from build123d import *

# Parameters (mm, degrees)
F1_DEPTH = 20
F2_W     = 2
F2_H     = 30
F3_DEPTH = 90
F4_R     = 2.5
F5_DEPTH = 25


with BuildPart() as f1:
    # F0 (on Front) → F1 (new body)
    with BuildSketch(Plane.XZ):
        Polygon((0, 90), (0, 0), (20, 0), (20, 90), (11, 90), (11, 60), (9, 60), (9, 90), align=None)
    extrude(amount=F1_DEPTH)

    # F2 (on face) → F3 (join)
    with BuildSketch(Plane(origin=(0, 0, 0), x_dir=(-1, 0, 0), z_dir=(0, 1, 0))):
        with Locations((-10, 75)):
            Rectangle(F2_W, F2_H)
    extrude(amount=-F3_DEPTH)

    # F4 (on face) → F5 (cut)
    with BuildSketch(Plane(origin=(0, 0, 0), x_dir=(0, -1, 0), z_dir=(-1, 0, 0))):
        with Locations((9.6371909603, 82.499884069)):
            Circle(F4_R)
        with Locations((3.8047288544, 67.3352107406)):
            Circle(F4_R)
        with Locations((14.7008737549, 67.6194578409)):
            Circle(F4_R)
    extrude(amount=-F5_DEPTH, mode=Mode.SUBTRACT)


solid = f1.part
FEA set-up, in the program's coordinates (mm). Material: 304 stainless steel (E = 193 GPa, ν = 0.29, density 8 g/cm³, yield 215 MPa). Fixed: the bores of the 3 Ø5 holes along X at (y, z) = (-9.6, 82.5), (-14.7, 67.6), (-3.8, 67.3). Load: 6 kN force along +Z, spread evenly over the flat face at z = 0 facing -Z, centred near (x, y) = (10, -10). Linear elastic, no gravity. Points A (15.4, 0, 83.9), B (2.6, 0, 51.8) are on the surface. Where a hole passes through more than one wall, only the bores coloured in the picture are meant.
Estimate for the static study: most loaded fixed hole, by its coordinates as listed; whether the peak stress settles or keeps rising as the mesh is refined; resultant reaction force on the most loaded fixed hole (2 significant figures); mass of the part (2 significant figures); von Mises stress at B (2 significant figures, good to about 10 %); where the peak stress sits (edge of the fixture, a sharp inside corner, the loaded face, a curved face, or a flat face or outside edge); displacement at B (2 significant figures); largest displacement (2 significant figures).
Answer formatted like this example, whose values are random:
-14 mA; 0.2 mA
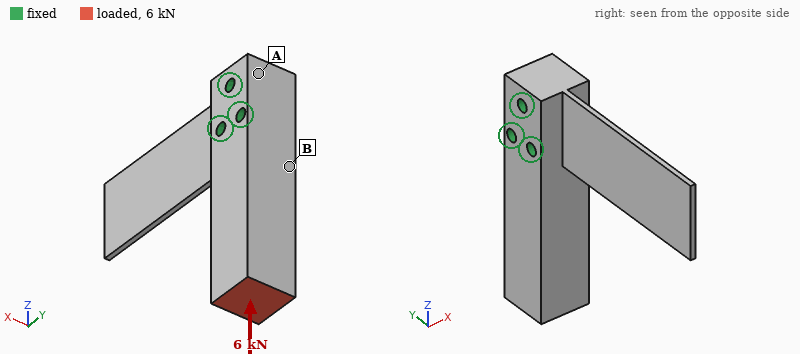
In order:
(-14.7, 67.6); keeps rising; 3.2 kN; 310 g; 15 MPa; edge of the fixture; 1.1 µm; 5.2 µm
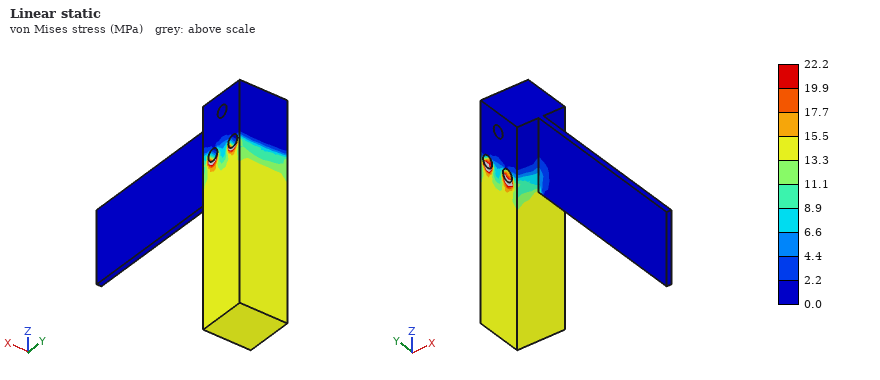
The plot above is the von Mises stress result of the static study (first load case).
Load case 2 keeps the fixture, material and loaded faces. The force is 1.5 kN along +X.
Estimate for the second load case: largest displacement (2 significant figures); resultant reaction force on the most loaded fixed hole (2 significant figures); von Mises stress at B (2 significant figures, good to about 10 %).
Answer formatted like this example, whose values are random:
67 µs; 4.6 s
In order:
61 µm; 840 N; 43 MPa
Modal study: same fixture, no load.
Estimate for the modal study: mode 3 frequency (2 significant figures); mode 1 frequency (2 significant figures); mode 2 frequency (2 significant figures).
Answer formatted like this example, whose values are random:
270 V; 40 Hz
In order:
2000 Hz; 330 Hz; 1600 Hz
